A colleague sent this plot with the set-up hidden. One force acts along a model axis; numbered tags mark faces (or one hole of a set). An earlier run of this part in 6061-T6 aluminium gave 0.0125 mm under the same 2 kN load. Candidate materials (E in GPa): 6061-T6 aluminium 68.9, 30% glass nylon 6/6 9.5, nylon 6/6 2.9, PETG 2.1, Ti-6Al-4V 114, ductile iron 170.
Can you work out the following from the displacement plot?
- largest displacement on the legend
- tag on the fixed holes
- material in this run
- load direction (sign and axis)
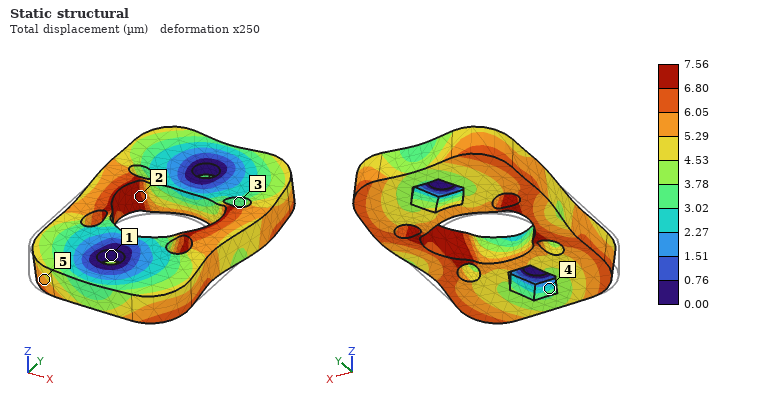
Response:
7.56 µm
1
Ti-6Al-4V
+Y
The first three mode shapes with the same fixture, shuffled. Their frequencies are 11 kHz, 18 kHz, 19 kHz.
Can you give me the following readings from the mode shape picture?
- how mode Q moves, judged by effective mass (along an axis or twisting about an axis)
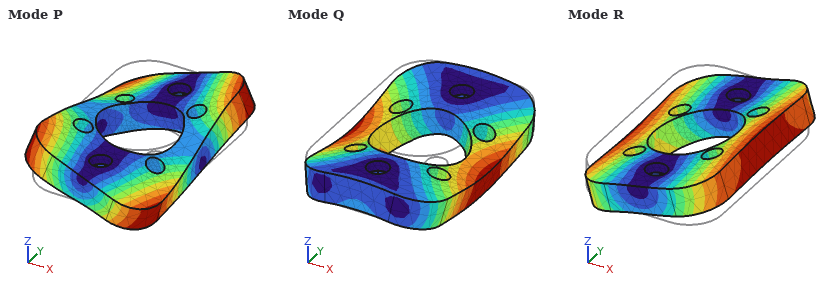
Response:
along Z
